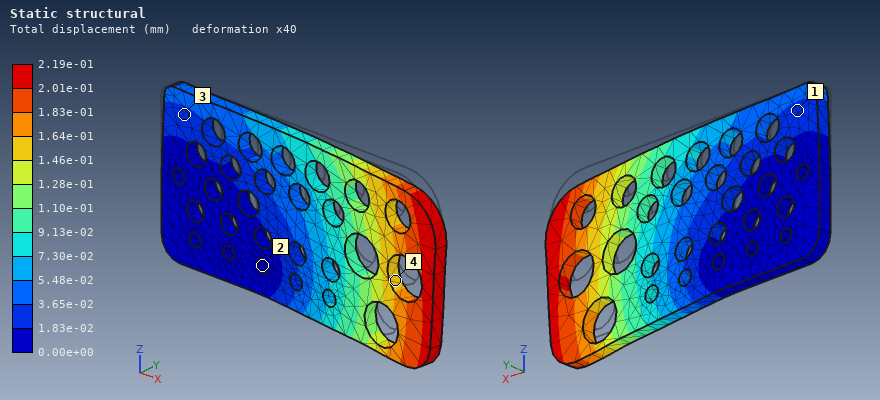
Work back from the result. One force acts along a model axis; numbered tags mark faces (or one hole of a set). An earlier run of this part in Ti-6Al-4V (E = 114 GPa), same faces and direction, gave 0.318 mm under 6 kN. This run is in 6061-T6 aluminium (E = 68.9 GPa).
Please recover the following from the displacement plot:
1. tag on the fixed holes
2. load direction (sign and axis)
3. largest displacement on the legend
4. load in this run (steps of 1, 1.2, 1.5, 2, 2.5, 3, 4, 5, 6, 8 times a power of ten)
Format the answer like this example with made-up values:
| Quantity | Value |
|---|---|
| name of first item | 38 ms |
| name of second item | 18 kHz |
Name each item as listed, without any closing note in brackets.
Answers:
| Quantity | Value |
|---|---|
| tag on the fixed holes | 2 |
| load direction | -Z |
| largest displacement on the legend | 2.19e-01 mm |
| load in this run | 2.5 kN |
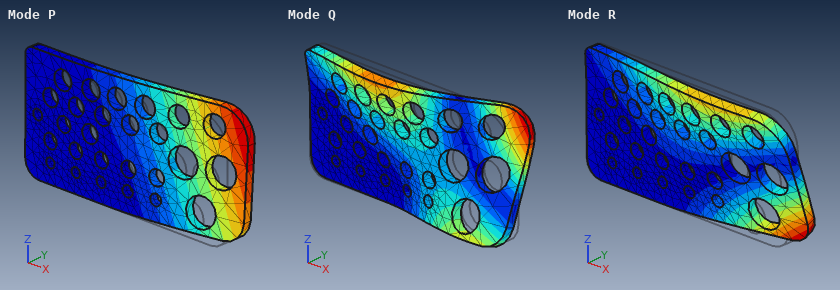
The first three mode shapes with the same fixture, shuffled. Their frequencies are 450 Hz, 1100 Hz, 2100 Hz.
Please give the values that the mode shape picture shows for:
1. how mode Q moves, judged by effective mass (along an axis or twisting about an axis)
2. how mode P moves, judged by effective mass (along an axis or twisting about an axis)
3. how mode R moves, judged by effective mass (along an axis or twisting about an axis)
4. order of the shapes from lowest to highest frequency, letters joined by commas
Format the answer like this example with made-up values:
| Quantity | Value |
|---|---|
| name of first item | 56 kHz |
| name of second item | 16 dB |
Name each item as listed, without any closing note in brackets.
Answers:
| Quantity | Value |
|---|---|
| how mode Q moves, judged by effective mass | along Y |
| how mode P moves, judged by effective mass | along Y |
| how mode R moves, judged by effective mass | twisting about X |
| order of the shapes from lowest to highest frequency, letters joined by commas | P, R, Q |
